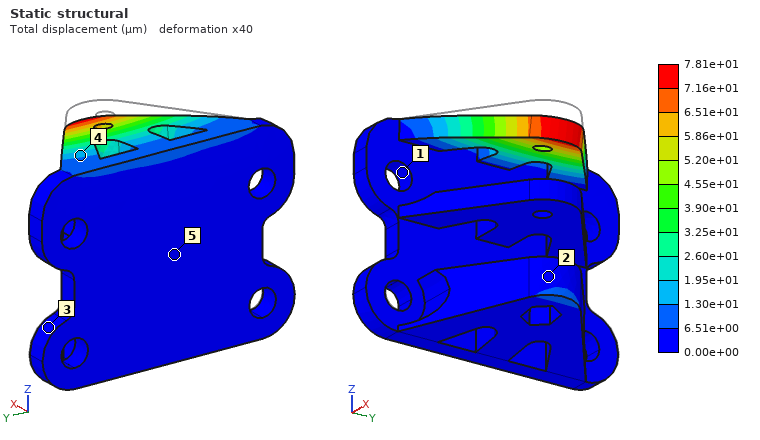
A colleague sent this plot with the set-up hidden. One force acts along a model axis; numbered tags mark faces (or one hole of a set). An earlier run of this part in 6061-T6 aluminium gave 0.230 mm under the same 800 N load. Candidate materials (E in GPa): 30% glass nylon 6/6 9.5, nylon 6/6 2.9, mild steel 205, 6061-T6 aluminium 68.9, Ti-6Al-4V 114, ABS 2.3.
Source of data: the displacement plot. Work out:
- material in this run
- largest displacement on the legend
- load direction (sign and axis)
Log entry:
mild steel
7.81e+01 µm
-Z
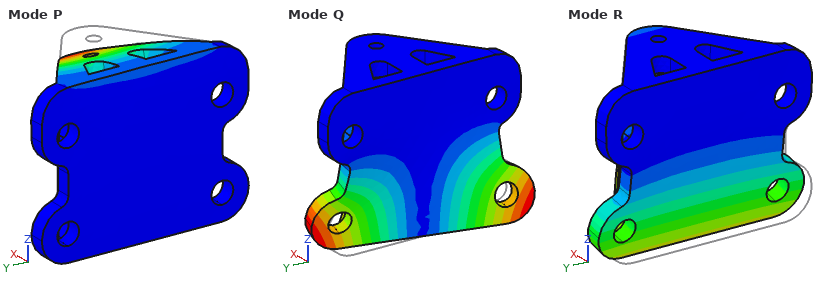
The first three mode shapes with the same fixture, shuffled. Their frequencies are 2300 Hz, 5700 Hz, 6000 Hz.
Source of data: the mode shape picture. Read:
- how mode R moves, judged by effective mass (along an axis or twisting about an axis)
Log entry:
along X
